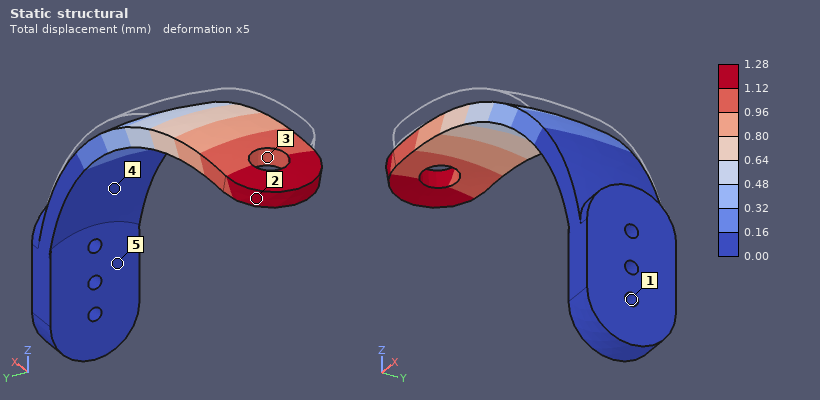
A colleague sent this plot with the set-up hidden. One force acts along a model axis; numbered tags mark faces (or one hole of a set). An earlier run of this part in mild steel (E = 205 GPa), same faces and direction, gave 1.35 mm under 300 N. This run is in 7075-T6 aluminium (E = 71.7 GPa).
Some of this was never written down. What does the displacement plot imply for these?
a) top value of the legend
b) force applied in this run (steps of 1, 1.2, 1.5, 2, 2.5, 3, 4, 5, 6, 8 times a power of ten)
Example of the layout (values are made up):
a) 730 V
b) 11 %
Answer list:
a) 1.28 mm
b) 100 N
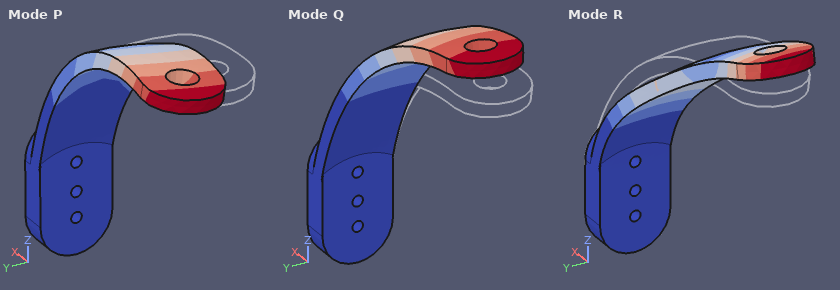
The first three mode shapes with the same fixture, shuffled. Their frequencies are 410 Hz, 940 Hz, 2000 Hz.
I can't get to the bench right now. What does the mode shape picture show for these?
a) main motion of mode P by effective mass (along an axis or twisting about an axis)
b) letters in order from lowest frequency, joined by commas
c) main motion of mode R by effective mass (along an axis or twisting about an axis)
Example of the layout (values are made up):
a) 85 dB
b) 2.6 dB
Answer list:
a) along Y
b) Q, P, R
c) along X
